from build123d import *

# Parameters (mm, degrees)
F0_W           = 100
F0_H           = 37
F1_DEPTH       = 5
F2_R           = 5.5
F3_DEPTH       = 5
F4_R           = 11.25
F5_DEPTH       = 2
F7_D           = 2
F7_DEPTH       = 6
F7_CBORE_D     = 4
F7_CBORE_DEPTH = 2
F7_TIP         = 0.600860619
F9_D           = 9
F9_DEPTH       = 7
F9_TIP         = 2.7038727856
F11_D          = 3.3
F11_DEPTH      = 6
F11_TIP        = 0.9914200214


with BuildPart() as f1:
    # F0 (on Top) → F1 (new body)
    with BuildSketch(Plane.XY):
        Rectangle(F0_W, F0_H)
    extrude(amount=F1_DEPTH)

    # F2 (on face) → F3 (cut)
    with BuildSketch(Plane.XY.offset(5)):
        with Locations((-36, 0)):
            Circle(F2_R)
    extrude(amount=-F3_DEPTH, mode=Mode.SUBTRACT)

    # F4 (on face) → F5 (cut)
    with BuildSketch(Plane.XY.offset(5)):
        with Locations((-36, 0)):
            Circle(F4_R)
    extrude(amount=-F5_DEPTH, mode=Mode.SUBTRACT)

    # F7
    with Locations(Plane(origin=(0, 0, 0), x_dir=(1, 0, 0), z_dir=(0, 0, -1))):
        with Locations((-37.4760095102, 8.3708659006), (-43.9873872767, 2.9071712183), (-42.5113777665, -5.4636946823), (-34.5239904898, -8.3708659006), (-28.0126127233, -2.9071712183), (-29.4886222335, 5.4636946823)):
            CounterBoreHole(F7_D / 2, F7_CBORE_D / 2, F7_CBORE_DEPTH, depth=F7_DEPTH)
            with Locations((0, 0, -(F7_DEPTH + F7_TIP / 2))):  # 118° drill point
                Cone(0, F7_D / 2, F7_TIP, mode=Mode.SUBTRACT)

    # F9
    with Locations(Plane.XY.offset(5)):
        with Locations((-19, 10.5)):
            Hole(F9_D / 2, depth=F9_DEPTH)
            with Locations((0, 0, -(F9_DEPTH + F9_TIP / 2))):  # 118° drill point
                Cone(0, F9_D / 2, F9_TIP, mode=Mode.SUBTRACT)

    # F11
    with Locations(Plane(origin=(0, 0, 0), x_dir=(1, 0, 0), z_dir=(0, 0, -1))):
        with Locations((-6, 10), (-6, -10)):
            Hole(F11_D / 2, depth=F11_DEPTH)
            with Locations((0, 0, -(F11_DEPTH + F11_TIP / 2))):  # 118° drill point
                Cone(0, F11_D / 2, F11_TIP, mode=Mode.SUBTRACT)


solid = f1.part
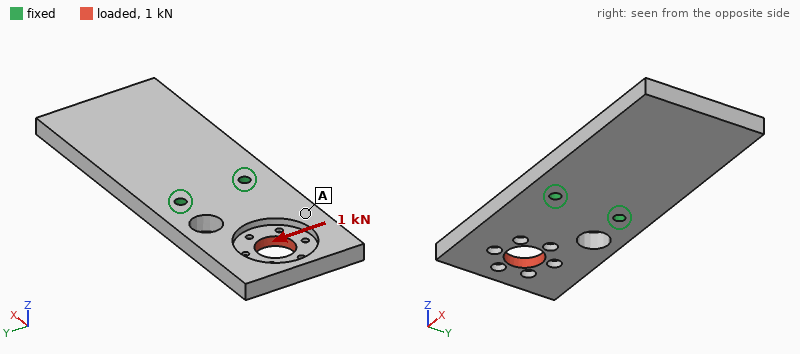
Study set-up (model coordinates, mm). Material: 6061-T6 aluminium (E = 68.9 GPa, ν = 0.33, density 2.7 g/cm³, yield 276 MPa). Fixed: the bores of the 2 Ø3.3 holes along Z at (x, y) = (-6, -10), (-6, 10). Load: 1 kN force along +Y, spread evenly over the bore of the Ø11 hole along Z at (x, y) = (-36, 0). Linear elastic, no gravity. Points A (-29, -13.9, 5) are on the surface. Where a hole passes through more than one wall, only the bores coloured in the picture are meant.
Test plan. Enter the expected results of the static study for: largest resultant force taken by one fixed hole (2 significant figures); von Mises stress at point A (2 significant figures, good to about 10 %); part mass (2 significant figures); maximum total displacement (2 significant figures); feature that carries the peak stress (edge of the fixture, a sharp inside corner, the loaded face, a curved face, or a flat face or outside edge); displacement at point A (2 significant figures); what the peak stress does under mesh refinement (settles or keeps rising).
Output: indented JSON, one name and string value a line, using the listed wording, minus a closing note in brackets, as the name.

{
  "largest resultant force taken by one fixed hole": "1.5 kN",
  "von Mises stress at point A": "6.6 MPa",
  "part mass": "45 g",
  "maximum total displacement": "39 µm",
  "feature that carries the peak stress": "edge of the fixture",
  "displacement at point A": "17 µm",
  "what the peak stress does under mesh refinement": "keeps rising"
}
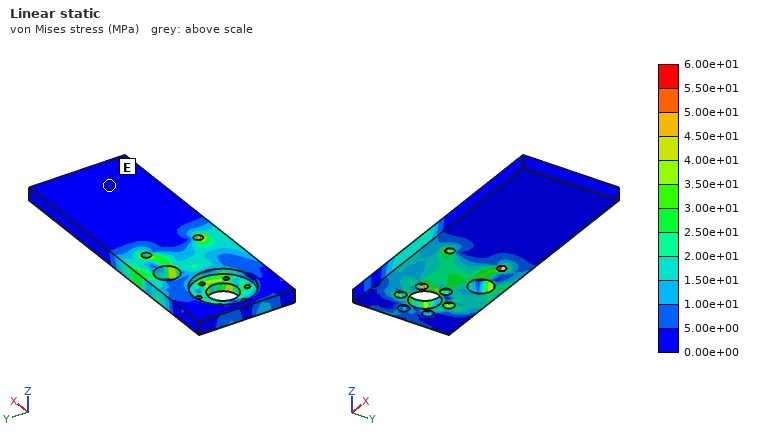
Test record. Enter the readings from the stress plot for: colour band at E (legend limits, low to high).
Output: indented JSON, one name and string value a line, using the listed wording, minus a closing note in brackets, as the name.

{
  "colour band at E": "0.00e+00 to 5.00e+00 MPa"
}
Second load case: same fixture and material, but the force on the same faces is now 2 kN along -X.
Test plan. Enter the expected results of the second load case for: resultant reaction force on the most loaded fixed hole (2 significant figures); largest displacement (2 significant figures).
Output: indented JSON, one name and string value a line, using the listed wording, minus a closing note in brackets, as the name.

{
  "resultant reaction force on the most loaded fixed hole": "1.0 kN",
  "largest displacement": "80 µm"
}
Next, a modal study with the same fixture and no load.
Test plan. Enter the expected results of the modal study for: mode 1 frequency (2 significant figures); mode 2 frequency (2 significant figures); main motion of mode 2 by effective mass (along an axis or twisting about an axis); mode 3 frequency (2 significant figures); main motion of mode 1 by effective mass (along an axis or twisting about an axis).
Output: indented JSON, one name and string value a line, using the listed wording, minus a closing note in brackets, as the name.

{
  "mode 1 frequency": "1300 Hz",
  "mode 2 frequency": "2100 Hz",
  "main motion of mode 2 by effective mass": "along Z",
  "mode 3 frequency": "4100 Hz",
  "main motion of mode 1 by effective mass": "along Z"
}
